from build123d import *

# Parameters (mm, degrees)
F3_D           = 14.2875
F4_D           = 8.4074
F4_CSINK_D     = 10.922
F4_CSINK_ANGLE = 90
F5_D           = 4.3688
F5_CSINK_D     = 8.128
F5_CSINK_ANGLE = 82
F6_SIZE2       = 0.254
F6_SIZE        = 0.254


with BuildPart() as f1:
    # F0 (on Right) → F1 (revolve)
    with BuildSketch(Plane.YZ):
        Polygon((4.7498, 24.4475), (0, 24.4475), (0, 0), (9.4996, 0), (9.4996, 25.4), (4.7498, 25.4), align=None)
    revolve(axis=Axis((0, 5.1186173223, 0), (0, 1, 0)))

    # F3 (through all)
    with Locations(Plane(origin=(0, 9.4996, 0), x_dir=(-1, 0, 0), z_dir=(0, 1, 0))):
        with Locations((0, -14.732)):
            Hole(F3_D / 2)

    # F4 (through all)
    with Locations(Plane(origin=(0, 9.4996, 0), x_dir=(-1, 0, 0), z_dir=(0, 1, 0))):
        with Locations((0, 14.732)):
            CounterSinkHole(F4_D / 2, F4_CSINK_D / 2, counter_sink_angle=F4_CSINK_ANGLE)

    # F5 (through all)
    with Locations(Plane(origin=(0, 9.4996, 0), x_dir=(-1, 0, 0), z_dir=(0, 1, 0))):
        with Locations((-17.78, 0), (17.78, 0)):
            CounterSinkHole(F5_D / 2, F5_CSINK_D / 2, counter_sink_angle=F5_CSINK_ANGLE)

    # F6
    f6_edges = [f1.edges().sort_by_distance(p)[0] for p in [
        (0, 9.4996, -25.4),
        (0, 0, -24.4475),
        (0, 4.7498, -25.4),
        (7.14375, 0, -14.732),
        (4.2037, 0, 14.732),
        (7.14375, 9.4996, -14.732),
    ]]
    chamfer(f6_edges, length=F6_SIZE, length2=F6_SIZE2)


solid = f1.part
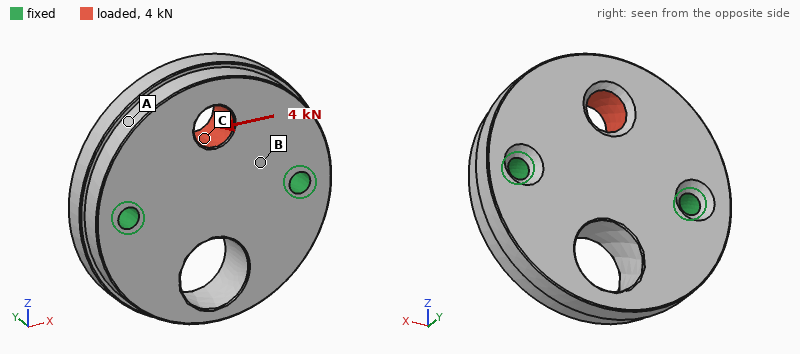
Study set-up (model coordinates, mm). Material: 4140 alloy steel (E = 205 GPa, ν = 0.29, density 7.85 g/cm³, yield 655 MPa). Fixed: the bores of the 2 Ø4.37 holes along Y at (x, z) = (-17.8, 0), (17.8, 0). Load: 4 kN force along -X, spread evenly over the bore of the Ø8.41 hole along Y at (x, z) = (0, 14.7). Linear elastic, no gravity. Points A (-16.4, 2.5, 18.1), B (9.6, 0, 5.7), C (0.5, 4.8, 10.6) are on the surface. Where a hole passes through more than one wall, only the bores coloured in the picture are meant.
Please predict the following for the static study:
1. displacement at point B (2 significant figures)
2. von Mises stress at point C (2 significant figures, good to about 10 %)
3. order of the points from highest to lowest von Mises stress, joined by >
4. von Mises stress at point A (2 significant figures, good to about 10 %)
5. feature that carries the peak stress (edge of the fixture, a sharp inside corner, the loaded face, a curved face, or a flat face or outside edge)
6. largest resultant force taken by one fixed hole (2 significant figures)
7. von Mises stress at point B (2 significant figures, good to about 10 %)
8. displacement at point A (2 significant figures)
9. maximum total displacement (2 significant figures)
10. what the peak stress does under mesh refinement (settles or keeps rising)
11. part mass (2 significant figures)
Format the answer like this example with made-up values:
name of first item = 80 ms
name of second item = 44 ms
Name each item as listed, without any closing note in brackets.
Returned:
displacement at point B = 1.1 µm
von Mises stress at point C = 39 MPa
order of the points from highest to lowest von Mises stress, joined by > = C > B > A
von Mises stress at point A = 7.2 MPa
feature that carries the peak stress = edge of the fixture
largest resultant force taken by one fixed hole = 2.5 kN
von Mises stress at point B = 20 MPa
displacement at point A = 2.9 µm
maximum total displacement = 4.0 µm
what the peak stress does under mesh refinement = keeps rising
part mass = 130 g
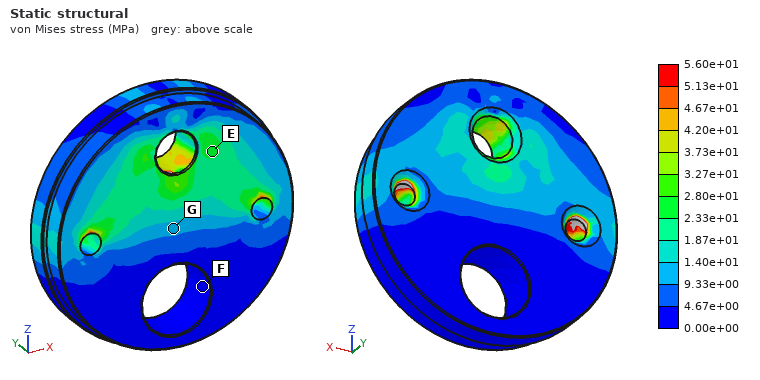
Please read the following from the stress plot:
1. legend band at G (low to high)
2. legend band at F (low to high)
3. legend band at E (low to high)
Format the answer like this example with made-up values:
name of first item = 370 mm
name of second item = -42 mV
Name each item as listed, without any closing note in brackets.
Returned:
legend band at G = 9.33e+00 to 1.40e+01 MPa
legend band at F = 0.00e+00 to 4.67e+00 MPa
legend band at E = 2.33e+01 to 2.80e+01 MPa
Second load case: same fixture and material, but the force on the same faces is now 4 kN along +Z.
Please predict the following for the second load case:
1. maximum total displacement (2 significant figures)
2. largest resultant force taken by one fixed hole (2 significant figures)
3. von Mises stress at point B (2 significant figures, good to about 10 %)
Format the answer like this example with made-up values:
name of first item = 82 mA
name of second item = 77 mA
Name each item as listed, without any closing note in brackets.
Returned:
maximum total displacement = 3.2 µm
largest resultant force taken by one fixed hole = 2.1 kN
von Mises stress at point B = 18 MPa
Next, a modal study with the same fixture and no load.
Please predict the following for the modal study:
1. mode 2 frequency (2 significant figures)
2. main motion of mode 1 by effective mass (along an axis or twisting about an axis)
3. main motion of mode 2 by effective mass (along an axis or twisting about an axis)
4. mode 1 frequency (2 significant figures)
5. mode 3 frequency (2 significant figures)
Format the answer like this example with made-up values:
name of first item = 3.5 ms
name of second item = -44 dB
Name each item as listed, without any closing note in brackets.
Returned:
mode 2 frequency = 13 kHz
main motion of mode 1 by effective mass = twisting about X
main motion of mode 2 by effective mass = along Y
mode 1 frequency = 9600 Hz
mode 3 frequency = 21 kHz
